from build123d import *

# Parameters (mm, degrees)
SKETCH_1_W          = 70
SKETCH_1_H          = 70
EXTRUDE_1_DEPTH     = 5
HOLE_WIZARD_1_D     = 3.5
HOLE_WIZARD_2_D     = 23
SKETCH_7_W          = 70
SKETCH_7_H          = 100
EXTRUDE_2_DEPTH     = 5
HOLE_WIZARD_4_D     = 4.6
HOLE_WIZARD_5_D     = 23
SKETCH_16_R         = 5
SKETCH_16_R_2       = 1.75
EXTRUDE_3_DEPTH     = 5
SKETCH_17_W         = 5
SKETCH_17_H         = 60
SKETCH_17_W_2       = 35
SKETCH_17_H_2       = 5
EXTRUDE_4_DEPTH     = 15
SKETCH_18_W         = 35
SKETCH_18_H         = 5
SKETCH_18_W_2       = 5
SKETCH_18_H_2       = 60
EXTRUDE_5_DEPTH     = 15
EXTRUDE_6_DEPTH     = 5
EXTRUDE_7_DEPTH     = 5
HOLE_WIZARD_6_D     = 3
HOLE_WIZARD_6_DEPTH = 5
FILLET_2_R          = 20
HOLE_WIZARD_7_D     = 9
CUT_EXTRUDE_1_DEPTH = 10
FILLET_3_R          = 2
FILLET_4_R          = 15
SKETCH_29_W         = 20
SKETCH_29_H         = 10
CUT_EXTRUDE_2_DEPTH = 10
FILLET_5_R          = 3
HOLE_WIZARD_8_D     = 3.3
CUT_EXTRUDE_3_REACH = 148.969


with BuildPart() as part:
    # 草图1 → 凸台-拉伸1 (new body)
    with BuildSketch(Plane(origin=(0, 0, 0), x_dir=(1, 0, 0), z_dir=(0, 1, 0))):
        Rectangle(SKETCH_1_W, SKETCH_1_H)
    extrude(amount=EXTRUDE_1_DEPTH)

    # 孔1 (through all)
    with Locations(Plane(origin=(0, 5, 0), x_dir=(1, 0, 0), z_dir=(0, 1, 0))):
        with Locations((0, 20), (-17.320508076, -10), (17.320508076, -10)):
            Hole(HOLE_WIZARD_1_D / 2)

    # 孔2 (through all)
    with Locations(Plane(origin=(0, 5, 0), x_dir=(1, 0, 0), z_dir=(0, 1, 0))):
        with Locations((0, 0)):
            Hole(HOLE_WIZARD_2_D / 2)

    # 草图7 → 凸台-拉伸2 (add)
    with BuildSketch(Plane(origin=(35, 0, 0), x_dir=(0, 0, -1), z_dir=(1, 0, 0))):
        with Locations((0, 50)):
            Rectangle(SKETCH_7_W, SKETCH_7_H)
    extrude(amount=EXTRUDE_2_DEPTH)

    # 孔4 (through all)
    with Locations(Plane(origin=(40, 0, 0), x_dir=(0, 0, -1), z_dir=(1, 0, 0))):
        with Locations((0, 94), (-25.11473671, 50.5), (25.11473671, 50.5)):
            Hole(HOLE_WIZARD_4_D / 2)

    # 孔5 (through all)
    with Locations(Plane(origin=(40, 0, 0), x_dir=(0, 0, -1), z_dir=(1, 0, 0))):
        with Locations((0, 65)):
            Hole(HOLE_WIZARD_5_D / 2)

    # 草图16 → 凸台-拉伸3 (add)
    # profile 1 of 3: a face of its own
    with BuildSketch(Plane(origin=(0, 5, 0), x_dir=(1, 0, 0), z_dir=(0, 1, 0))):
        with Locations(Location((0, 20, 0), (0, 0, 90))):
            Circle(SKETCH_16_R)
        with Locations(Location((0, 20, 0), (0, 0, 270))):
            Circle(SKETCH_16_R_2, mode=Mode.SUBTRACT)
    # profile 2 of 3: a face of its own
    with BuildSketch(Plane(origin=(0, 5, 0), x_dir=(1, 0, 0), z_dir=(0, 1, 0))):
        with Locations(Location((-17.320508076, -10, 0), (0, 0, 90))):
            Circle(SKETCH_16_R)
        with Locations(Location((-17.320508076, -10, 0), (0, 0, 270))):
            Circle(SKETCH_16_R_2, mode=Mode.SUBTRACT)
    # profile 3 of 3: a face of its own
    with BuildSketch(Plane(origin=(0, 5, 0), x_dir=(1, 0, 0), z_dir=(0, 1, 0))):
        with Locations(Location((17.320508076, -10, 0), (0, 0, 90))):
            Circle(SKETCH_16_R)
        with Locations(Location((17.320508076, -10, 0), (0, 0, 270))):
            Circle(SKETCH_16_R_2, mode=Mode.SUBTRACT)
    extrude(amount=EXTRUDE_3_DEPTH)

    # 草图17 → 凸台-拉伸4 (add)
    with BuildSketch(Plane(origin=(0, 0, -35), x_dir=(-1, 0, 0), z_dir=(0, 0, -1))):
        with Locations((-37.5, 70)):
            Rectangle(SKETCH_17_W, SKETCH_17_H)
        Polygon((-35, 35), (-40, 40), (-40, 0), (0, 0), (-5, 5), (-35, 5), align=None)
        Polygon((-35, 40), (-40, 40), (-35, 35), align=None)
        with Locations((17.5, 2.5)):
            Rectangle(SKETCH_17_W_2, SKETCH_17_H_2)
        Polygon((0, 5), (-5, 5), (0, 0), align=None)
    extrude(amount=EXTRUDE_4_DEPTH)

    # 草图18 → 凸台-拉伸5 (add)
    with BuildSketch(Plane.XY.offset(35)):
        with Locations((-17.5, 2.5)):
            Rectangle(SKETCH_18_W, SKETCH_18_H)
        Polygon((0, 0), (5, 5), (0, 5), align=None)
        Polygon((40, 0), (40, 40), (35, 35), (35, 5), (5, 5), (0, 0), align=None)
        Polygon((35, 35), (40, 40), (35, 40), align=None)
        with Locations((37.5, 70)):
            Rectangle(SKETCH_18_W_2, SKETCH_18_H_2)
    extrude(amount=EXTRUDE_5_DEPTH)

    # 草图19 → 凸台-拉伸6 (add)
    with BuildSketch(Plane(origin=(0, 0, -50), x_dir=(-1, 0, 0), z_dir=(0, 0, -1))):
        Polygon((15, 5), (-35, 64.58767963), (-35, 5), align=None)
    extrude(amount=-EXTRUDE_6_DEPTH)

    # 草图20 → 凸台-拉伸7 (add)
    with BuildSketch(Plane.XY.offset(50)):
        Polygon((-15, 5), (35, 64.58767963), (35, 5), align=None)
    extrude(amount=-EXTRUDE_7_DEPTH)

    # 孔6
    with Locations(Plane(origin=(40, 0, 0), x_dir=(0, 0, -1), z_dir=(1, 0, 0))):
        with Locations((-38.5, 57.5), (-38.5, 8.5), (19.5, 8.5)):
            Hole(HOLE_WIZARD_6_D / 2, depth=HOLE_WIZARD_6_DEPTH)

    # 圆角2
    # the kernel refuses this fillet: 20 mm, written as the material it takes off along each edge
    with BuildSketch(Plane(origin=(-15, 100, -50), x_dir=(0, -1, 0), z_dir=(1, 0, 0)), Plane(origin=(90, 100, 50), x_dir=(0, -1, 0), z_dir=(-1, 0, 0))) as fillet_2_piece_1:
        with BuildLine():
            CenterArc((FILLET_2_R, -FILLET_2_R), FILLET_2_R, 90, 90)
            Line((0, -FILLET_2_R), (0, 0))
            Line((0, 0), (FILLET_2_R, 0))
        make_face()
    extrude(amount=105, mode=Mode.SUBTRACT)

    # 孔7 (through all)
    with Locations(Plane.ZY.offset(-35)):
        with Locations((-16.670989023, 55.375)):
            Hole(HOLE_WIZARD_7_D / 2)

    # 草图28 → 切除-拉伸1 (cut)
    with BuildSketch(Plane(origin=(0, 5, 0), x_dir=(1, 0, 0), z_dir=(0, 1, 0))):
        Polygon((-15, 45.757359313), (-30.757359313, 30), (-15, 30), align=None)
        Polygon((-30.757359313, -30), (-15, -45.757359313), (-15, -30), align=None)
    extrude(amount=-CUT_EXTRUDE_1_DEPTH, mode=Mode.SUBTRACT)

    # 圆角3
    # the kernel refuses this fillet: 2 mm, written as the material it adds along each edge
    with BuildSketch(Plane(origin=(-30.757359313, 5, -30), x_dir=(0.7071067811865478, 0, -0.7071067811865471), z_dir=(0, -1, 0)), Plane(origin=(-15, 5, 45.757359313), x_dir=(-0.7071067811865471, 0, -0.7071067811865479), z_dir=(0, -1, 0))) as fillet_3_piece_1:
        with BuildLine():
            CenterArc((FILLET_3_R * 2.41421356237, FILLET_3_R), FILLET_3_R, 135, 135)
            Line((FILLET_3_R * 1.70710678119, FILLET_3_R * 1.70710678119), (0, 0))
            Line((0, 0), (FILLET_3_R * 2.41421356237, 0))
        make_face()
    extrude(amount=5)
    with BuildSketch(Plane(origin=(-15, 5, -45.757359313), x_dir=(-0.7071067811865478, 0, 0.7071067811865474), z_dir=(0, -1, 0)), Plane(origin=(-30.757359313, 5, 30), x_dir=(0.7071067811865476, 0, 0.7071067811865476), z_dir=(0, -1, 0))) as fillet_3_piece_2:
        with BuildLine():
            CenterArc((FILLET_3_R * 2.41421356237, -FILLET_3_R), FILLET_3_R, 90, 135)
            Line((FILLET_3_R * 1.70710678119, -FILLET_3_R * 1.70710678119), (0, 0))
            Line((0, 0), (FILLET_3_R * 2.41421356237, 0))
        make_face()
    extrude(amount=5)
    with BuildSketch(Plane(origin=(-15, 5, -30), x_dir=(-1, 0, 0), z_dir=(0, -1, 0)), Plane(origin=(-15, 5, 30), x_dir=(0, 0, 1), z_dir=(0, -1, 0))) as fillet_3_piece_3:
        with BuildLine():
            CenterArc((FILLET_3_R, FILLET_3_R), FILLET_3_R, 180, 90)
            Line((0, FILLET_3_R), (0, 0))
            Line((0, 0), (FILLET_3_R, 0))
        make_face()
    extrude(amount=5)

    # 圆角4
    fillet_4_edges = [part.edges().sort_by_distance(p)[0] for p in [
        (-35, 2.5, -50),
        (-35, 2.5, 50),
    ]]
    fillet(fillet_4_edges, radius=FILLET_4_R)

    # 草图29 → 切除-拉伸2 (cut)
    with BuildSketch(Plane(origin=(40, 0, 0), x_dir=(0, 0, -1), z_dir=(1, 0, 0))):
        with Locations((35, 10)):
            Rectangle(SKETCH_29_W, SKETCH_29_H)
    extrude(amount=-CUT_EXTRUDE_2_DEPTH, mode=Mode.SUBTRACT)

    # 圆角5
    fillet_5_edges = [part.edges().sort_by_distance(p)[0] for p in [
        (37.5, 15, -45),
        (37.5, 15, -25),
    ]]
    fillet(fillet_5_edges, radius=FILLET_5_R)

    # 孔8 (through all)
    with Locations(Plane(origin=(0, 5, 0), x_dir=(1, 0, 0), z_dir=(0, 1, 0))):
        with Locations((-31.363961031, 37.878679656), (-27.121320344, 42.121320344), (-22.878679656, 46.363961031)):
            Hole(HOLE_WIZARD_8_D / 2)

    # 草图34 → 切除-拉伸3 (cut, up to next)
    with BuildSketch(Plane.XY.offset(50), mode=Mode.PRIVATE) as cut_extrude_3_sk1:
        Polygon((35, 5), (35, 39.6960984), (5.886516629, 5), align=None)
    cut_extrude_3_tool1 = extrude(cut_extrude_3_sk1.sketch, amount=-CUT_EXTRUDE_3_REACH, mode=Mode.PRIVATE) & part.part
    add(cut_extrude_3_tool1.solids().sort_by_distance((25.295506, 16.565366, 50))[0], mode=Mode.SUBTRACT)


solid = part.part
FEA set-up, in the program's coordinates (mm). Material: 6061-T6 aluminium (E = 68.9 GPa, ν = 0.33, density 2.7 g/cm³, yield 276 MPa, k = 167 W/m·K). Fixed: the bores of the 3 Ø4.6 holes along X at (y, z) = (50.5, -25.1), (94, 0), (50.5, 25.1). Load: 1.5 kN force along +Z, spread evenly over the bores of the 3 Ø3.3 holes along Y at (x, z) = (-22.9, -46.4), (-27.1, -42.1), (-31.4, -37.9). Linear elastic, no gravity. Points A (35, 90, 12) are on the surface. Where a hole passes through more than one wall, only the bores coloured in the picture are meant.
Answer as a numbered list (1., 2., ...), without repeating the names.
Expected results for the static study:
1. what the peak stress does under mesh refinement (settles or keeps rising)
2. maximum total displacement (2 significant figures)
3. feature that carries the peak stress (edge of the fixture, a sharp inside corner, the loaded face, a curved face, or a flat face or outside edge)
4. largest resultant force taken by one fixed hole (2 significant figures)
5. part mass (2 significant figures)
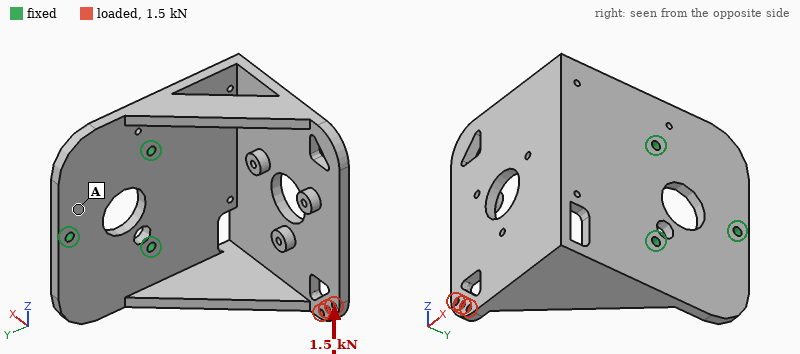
1. keeps rising
2. 1.2 mm
3. edge of the fixture
4. 2.1 kN
5. 240 g
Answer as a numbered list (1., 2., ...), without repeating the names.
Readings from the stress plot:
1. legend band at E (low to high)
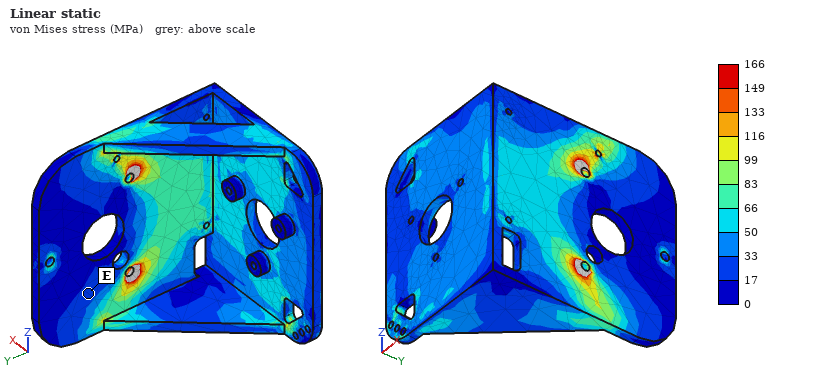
1. 17 to 33 MPa
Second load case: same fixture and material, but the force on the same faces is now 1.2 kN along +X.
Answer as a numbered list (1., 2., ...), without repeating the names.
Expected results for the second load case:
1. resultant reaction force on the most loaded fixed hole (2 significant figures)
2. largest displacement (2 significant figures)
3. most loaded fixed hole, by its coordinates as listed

1. 1.6 kN
2. 1.3 mm
3. (50.5, -25.1)
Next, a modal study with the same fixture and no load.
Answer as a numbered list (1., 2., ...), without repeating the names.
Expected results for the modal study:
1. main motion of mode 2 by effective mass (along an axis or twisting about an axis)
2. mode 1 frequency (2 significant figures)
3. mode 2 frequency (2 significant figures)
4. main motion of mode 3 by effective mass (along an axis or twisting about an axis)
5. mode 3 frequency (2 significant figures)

1. along Z
2. 580 Hz
3. 770 Hz
4. along X
5. 1800 Hz
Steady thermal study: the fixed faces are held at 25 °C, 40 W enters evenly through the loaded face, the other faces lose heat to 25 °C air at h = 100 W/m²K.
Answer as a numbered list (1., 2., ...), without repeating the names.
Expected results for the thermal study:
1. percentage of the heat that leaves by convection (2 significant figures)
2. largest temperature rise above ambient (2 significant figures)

1. 75 %
2. 71 K
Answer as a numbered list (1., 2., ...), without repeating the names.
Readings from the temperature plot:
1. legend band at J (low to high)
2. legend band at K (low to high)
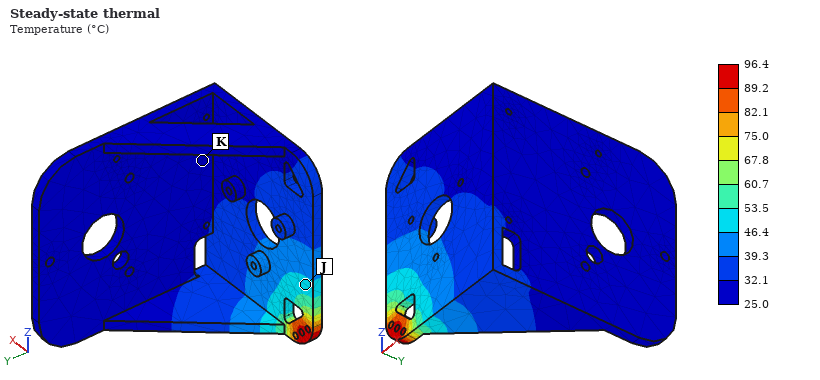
1. 46.4 to 53.5 °C
2. 25.0 to 32.1 °C
